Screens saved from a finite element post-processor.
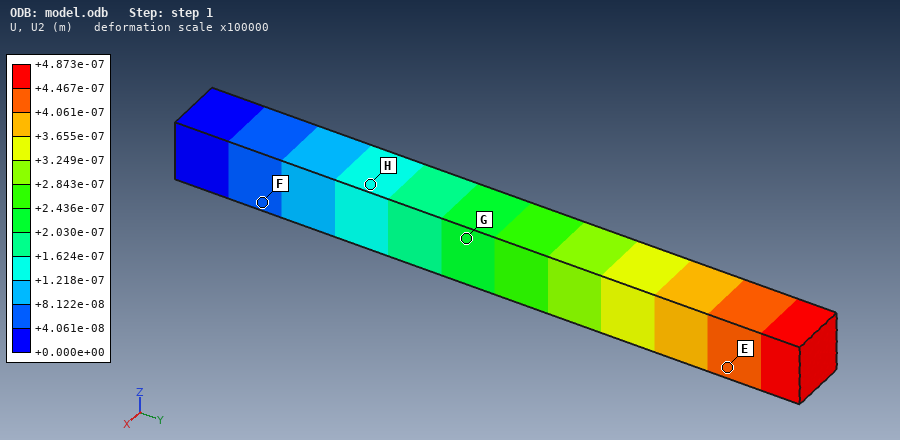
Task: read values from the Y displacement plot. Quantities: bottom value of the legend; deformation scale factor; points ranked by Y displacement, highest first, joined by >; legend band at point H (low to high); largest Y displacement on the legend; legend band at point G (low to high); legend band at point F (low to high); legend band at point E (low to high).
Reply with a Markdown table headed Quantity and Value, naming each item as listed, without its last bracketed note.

| Quantity | Value |
|---|---|
| bottom value of the legend | +0.000e+00 m |
| deformation scale factor | 100000 |
| points ranked by Y displacement, highest first, joined by > | E > G > H > F |
| legend band at point H | +1.218e-07 to +1.624e-07 m |
| largest Y displacement on the legend | +4.873e-07 m |
| legend band at point G | +2.030e-07 to +2.436e-07 m |
| legend band at point F | +4.061e-08 to +8.122e-08 m |
| legend band at point E | +4.061e-07 to +4.467e-07 m |
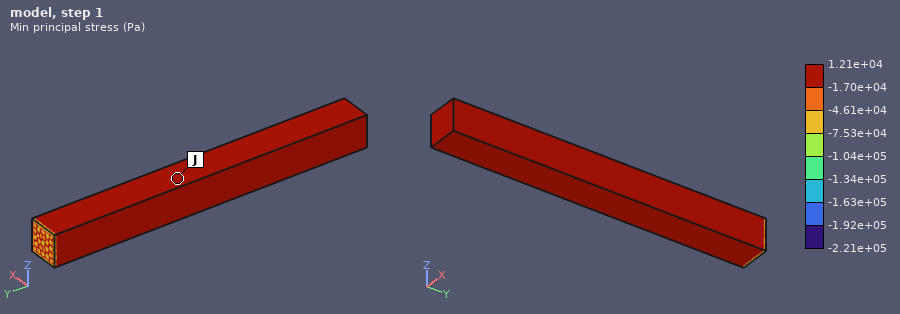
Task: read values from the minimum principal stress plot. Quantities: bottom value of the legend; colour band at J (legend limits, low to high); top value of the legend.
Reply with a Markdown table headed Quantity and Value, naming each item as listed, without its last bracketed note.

| Quantity | Value |
|---|---|
| bottom value of the legend | -2.21e+05 Pa |
| colour band at J | -1.70e+04 to 1.21e+04 Pa |
| top value of the legend | 1.21e+04 Pa |
